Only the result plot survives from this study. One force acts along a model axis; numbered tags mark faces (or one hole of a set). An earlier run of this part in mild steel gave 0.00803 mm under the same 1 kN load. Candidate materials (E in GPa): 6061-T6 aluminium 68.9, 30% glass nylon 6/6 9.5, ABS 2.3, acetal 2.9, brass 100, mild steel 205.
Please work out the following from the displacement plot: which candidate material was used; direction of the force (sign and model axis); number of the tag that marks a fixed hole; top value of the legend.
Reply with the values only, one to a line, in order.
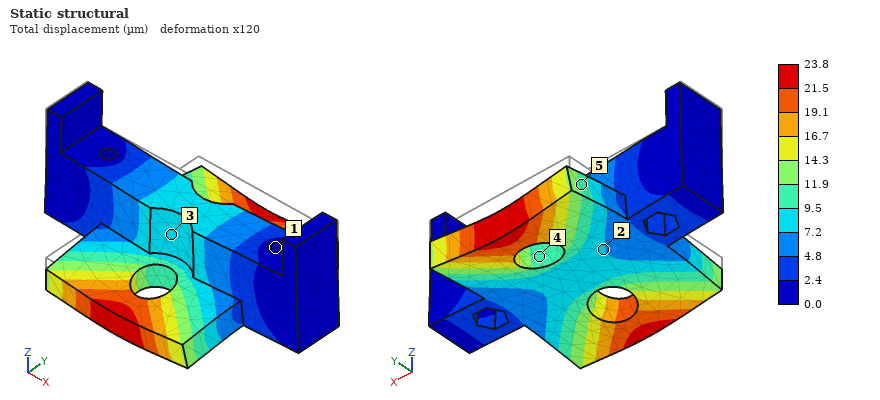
6061-T6 aluminium
-Z
1
23.8 µm
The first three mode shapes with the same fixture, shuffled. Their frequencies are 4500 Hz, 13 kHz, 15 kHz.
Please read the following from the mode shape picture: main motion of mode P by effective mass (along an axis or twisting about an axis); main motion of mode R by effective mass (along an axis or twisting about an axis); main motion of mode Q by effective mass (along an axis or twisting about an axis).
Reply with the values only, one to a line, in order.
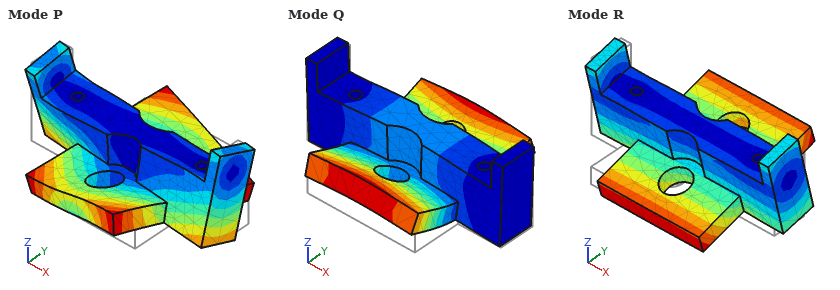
twisting about Z
along Y
along Z
